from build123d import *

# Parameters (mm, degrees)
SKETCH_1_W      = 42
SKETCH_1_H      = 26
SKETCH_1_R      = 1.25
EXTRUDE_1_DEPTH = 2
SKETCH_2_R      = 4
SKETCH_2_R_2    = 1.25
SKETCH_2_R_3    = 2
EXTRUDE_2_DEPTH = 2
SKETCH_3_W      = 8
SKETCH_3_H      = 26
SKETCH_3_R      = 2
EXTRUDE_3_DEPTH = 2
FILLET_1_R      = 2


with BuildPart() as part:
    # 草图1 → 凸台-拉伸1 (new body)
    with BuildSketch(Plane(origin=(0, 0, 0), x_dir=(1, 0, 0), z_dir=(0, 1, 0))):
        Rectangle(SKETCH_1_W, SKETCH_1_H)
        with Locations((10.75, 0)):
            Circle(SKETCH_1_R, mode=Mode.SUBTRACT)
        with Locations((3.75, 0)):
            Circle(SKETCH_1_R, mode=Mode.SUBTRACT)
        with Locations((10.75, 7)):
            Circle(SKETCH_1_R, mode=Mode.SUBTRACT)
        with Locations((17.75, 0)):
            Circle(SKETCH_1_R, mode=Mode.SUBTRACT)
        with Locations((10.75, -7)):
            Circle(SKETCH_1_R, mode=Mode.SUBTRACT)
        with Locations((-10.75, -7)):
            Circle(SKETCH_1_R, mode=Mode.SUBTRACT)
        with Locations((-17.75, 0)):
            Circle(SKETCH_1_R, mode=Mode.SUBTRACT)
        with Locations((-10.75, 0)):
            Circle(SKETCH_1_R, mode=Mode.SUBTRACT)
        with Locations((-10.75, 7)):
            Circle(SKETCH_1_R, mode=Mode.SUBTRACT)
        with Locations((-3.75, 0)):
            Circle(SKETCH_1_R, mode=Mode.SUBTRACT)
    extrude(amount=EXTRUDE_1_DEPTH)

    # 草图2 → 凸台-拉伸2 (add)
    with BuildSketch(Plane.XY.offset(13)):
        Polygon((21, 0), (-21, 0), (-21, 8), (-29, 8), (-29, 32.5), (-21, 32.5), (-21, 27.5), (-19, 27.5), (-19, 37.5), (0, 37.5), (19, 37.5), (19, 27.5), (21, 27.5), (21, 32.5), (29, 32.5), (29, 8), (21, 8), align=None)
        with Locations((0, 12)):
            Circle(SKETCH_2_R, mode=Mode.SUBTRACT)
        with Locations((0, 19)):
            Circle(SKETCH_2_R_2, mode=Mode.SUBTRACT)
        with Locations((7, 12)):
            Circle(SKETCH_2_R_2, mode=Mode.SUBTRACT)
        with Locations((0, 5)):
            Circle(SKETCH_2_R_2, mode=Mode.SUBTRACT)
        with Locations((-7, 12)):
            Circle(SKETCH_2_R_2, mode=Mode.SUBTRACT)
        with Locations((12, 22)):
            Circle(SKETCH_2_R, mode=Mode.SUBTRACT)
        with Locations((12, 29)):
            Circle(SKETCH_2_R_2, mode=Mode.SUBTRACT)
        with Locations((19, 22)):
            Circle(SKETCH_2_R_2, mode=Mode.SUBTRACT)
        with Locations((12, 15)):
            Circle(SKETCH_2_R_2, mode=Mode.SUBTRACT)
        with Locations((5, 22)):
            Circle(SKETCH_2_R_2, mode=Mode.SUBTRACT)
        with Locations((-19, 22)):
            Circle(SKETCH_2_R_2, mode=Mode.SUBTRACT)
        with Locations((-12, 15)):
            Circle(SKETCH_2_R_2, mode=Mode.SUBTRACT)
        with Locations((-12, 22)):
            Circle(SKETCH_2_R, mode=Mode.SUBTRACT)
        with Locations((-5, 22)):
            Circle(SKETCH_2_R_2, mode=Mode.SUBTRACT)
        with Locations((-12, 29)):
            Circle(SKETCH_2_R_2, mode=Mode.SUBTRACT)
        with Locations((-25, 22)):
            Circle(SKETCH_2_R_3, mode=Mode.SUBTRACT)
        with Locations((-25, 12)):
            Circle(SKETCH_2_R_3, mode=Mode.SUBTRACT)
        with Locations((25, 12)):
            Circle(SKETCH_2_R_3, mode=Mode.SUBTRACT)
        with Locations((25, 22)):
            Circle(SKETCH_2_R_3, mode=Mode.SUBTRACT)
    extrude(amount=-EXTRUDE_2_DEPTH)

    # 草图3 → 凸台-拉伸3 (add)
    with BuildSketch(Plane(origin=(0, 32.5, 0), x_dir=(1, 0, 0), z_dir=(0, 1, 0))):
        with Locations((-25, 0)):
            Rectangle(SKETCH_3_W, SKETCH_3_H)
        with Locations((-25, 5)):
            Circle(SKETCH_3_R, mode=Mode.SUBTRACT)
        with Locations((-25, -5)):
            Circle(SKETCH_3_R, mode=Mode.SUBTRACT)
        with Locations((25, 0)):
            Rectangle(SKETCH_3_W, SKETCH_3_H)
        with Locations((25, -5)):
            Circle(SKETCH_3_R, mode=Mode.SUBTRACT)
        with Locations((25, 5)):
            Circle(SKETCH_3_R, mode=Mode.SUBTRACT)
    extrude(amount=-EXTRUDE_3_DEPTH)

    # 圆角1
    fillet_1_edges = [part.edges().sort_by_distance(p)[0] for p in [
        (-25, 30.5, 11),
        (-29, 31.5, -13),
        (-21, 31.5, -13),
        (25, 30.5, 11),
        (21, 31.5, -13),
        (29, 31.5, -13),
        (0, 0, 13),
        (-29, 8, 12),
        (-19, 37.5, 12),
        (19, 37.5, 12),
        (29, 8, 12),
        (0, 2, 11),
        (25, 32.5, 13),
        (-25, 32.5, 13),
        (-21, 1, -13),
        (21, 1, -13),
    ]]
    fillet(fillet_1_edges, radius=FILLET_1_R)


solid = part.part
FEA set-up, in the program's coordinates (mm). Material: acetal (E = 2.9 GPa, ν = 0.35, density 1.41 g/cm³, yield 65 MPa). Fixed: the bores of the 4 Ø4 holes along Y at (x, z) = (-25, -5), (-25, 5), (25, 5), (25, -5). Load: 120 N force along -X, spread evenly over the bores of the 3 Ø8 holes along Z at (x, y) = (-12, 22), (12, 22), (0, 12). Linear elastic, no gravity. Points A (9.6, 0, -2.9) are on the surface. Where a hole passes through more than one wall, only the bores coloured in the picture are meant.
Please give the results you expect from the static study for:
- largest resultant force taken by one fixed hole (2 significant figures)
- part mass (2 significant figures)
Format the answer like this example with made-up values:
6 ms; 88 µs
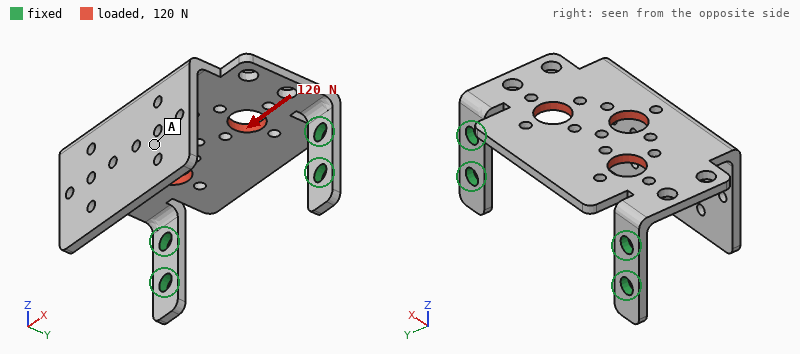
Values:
72 N; 8.3 g
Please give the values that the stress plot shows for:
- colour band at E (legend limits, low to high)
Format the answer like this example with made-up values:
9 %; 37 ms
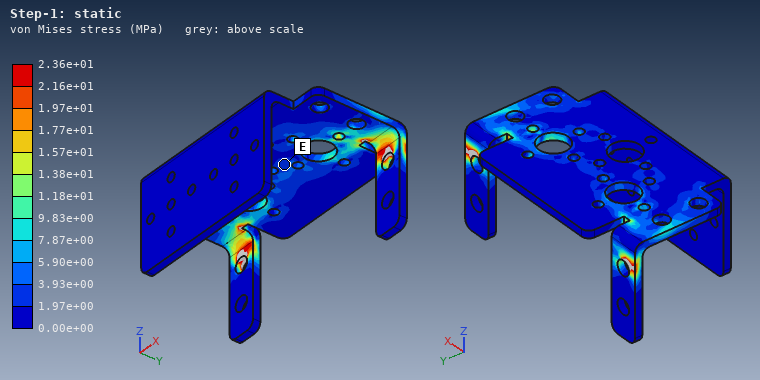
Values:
1.97e+00 to 3.93e+00 MPa
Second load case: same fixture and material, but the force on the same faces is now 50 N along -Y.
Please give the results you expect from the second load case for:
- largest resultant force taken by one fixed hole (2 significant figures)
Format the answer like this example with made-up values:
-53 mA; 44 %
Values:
26 N
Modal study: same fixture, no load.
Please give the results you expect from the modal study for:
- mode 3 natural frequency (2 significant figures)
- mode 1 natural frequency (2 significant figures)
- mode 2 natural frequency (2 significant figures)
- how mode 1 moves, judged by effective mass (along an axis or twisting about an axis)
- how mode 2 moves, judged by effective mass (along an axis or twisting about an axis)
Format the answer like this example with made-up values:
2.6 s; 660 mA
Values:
470 Hz; 120 Hz; 360 Hz; along Z; along X
